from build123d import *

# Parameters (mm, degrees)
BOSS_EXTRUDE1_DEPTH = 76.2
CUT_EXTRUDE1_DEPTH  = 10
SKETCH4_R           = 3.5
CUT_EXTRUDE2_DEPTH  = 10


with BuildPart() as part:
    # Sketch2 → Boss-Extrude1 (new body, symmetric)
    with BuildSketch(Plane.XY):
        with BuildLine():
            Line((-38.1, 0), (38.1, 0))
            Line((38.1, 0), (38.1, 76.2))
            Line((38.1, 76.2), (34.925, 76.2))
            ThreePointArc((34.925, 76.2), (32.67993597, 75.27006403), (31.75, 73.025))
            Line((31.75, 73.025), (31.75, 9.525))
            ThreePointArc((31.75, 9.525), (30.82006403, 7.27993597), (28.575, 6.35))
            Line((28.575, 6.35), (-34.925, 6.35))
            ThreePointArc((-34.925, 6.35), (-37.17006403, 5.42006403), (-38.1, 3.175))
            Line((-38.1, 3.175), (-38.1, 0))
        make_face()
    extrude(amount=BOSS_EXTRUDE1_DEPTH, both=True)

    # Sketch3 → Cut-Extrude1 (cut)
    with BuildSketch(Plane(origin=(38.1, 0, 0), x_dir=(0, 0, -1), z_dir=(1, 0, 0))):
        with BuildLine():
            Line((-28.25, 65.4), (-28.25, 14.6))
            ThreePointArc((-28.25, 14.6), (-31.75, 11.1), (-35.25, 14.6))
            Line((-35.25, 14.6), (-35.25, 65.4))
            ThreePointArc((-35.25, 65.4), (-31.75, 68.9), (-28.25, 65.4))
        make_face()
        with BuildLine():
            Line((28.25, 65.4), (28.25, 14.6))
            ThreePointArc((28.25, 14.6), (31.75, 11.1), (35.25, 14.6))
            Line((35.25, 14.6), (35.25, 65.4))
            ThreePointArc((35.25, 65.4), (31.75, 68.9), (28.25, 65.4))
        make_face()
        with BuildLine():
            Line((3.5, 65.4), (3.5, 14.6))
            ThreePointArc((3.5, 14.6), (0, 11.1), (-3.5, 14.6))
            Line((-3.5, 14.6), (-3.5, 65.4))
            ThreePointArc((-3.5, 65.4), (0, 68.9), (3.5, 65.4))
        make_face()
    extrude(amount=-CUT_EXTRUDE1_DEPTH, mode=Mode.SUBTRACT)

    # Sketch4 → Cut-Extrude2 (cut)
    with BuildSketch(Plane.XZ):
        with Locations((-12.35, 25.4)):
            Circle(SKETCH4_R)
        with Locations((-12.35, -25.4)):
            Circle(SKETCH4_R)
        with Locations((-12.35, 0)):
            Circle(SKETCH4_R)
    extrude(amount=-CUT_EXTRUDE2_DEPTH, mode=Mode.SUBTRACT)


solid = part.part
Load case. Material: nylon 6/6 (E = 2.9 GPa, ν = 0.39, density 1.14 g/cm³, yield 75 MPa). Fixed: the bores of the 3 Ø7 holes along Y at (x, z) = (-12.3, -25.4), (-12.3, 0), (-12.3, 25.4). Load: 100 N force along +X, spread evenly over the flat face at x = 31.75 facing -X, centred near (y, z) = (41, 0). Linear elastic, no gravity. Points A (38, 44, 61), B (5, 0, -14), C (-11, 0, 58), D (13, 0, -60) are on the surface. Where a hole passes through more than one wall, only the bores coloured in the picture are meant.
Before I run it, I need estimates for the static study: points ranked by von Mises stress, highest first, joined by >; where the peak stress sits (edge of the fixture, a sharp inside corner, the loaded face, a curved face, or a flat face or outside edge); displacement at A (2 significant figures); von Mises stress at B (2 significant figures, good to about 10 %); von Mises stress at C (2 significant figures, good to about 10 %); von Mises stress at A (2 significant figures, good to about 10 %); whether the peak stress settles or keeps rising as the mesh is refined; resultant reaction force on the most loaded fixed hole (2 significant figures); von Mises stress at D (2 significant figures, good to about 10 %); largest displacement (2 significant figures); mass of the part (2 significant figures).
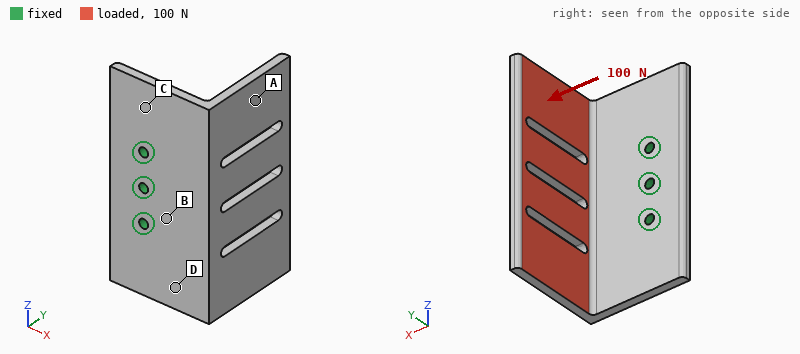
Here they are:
B > D > C > A
edge of the fixture
1.1 mm
3.9 MPa
1.8 MPa
0.75 MPa
keeps rising
43 N
2.9 MPa
2.0 mm
150 g
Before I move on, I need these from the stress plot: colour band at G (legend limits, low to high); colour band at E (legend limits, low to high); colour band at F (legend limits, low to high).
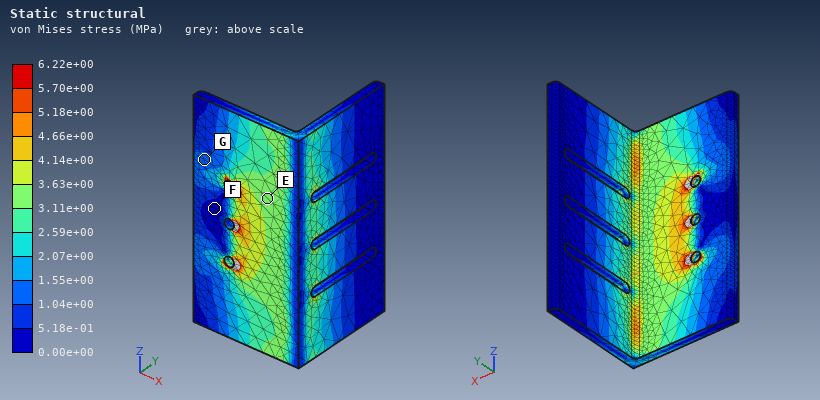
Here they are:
1.04e+00 to 1.55e+00 MPa
3.11e+00 to 3.63e+00 MPa
0.00e+00 to 5.18e-01 MPa
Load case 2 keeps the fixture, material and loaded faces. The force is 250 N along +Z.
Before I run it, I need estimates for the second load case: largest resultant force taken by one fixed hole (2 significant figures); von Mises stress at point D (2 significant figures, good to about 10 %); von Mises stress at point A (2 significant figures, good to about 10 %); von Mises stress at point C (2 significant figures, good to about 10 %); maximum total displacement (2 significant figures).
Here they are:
260 N
1.7 MPa
1.5 MPa
3.1 MPa
2.0 mm
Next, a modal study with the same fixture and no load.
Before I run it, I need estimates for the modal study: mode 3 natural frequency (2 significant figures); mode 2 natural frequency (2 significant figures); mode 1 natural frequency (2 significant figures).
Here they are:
380 Hz
200 Hz
150 Hz
